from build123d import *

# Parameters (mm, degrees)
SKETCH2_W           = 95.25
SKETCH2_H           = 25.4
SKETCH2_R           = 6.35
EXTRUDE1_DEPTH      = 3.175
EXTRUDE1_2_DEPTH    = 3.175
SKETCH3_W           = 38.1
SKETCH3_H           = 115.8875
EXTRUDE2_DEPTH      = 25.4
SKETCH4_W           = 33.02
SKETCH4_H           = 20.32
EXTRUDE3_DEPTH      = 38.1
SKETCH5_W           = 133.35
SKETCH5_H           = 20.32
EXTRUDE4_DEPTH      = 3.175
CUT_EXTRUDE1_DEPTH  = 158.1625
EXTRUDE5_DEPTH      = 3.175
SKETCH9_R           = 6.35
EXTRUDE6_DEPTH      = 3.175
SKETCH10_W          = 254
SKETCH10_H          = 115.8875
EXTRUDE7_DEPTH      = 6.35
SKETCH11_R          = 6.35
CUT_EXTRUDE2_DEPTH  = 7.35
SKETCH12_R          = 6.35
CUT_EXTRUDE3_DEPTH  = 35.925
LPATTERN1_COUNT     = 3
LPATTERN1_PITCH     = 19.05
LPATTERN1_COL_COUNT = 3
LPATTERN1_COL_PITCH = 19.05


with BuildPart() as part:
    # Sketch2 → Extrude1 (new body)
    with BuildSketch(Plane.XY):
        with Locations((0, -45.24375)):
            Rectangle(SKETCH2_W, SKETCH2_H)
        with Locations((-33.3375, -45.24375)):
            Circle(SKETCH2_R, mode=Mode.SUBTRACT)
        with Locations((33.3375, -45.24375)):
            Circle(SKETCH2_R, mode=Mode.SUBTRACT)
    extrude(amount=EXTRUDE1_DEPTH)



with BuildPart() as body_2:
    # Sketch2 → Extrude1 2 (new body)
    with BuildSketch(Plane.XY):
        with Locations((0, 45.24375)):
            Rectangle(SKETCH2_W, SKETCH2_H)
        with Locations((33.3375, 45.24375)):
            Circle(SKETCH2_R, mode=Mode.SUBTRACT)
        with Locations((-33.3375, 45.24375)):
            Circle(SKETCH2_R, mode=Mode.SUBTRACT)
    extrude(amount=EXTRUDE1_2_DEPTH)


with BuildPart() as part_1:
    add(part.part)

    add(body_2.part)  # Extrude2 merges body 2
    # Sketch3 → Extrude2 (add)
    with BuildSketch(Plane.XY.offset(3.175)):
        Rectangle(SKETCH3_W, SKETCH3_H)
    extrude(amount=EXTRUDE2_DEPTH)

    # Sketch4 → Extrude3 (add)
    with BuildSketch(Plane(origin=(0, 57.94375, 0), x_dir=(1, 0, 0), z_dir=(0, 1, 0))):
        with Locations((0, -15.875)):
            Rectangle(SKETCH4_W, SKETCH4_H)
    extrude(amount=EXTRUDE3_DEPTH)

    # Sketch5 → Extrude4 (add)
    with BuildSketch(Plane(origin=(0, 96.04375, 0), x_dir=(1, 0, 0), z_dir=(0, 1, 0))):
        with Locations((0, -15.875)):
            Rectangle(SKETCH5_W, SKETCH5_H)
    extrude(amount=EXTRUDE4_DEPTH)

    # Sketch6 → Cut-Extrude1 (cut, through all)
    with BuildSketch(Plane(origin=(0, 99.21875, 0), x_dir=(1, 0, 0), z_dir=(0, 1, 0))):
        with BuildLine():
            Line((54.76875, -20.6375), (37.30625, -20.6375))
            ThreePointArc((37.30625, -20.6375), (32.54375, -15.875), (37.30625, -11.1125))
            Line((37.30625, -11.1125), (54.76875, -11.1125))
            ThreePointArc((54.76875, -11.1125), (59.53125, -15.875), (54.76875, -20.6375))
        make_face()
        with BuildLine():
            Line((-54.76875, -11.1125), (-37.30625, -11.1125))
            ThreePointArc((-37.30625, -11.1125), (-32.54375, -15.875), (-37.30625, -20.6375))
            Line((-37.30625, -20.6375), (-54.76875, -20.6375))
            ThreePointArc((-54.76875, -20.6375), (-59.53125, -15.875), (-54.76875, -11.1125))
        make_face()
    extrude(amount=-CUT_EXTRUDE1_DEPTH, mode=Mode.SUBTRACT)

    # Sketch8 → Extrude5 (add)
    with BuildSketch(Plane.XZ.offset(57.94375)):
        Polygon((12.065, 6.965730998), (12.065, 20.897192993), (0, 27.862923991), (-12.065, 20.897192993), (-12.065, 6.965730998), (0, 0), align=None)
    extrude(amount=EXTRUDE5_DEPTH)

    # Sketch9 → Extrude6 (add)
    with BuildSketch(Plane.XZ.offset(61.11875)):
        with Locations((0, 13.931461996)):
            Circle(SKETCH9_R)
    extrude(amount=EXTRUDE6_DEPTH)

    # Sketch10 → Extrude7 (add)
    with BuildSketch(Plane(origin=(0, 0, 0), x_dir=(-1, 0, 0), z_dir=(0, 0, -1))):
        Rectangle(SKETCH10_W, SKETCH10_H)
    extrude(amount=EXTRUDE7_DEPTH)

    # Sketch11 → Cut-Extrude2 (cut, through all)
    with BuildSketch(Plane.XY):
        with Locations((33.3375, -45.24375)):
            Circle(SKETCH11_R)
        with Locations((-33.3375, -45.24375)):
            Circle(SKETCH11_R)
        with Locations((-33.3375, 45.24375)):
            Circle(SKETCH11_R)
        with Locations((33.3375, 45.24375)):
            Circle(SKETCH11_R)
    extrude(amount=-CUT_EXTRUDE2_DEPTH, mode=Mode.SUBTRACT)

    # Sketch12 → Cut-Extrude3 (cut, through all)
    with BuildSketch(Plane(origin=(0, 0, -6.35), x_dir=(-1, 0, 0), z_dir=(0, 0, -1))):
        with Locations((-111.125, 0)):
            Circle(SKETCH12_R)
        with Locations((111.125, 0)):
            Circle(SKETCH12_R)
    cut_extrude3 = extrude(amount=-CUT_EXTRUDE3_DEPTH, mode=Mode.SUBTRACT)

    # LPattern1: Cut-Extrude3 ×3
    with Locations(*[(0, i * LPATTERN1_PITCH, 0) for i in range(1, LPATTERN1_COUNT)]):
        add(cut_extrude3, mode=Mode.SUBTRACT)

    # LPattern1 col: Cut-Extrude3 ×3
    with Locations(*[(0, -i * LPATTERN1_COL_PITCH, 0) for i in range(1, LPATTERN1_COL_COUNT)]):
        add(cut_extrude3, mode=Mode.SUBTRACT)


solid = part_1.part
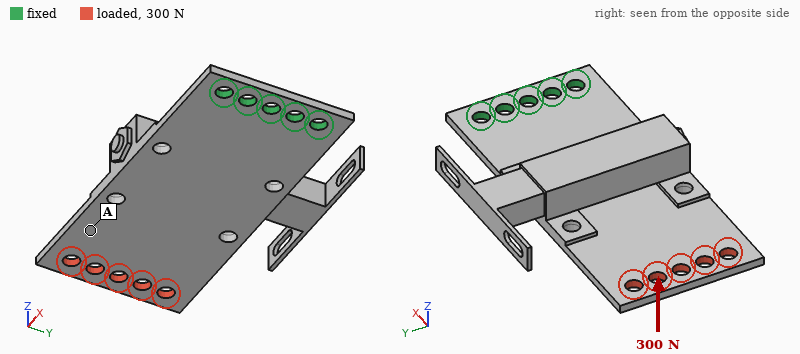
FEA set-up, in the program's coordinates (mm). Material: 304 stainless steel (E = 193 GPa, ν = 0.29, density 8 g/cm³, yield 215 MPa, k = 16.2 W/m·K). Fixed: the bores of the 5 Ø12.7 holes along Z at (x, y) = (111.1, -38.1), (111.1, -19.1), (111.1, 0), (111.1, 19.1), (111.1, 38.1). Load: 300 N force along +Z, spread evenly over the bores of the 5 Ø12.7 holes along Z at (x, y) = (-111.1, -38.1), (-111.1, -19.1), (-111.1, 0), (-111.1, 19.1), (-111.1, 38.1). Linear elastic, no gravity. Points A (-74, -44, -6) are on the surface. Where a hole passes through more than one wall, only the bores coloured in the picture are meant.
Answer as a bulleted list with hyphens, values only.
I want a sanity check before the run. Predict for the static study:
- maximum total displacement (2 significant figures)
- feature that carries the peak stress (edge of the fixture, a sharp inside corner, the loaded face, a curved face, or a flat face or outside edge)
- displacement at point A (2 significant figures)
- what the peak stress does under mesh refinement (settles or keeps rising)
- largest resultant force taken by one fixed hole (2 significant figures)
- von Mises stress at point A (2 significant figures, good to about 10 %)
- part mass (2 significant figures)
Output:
- 1.8 mm
- edge of the fixture
- 1.3 mm
- keeps rising
- 160 N
- 14 MPa
- 2.7 kg
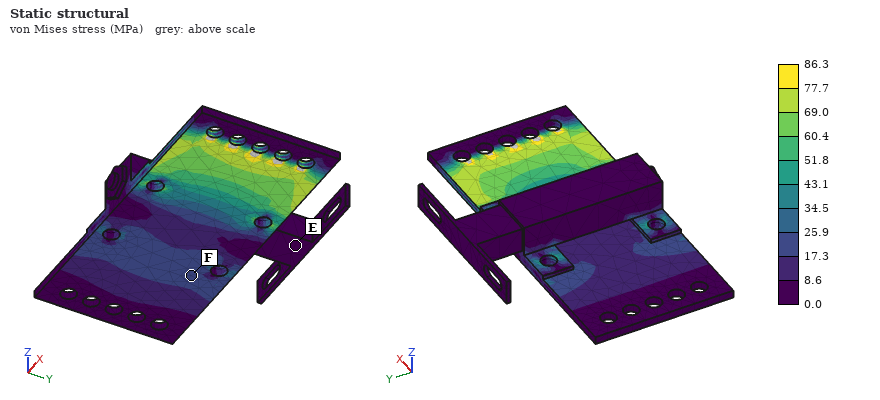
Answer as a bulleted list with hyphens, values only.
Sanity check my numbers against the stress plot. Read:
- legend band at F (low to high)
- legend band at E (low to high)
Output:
- 17.3 to 25.9 MPa
- 0.0 to 8.6 MPa
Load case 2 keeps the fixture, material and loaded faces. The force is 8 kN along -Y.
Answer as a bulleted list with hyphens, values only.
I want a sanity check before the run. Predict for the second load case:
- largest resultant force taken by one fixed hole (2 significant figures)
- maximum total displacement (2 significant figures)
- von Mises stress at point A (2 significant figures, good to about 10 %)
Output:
- 19 kN
- 0.27 mm
- 14 MPa
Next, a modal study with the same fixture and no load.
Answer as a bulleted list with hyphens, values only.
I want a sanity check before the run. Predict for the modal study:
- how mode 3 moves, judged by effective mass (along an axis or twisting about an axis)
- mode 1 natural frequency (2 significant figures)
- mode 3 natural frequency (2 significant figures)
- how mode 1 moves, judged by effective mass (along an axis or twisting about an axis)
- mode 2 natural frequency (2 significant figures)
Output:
- along Z
- 88 Hz
- 550 Hz
- along Z
- 330 Hz
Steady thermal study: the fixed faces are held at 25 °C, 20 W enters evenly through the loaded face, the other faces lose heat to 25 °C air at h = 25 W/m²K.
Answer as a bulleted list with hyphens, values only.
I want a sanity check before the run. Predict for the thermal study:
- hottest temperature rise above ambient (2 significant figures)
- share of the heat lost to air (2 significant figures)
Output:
- 68 K
- 99 %
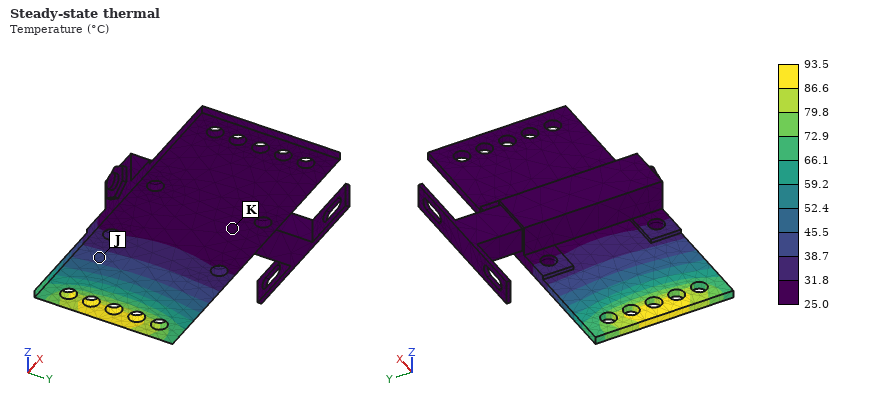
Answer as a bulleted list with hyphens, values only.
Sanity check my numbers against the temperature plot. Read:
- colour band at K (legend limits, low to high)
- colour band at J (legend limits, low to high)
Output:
- 25.0 to 31.8 °C
- 38.7 to 45.5 °C
